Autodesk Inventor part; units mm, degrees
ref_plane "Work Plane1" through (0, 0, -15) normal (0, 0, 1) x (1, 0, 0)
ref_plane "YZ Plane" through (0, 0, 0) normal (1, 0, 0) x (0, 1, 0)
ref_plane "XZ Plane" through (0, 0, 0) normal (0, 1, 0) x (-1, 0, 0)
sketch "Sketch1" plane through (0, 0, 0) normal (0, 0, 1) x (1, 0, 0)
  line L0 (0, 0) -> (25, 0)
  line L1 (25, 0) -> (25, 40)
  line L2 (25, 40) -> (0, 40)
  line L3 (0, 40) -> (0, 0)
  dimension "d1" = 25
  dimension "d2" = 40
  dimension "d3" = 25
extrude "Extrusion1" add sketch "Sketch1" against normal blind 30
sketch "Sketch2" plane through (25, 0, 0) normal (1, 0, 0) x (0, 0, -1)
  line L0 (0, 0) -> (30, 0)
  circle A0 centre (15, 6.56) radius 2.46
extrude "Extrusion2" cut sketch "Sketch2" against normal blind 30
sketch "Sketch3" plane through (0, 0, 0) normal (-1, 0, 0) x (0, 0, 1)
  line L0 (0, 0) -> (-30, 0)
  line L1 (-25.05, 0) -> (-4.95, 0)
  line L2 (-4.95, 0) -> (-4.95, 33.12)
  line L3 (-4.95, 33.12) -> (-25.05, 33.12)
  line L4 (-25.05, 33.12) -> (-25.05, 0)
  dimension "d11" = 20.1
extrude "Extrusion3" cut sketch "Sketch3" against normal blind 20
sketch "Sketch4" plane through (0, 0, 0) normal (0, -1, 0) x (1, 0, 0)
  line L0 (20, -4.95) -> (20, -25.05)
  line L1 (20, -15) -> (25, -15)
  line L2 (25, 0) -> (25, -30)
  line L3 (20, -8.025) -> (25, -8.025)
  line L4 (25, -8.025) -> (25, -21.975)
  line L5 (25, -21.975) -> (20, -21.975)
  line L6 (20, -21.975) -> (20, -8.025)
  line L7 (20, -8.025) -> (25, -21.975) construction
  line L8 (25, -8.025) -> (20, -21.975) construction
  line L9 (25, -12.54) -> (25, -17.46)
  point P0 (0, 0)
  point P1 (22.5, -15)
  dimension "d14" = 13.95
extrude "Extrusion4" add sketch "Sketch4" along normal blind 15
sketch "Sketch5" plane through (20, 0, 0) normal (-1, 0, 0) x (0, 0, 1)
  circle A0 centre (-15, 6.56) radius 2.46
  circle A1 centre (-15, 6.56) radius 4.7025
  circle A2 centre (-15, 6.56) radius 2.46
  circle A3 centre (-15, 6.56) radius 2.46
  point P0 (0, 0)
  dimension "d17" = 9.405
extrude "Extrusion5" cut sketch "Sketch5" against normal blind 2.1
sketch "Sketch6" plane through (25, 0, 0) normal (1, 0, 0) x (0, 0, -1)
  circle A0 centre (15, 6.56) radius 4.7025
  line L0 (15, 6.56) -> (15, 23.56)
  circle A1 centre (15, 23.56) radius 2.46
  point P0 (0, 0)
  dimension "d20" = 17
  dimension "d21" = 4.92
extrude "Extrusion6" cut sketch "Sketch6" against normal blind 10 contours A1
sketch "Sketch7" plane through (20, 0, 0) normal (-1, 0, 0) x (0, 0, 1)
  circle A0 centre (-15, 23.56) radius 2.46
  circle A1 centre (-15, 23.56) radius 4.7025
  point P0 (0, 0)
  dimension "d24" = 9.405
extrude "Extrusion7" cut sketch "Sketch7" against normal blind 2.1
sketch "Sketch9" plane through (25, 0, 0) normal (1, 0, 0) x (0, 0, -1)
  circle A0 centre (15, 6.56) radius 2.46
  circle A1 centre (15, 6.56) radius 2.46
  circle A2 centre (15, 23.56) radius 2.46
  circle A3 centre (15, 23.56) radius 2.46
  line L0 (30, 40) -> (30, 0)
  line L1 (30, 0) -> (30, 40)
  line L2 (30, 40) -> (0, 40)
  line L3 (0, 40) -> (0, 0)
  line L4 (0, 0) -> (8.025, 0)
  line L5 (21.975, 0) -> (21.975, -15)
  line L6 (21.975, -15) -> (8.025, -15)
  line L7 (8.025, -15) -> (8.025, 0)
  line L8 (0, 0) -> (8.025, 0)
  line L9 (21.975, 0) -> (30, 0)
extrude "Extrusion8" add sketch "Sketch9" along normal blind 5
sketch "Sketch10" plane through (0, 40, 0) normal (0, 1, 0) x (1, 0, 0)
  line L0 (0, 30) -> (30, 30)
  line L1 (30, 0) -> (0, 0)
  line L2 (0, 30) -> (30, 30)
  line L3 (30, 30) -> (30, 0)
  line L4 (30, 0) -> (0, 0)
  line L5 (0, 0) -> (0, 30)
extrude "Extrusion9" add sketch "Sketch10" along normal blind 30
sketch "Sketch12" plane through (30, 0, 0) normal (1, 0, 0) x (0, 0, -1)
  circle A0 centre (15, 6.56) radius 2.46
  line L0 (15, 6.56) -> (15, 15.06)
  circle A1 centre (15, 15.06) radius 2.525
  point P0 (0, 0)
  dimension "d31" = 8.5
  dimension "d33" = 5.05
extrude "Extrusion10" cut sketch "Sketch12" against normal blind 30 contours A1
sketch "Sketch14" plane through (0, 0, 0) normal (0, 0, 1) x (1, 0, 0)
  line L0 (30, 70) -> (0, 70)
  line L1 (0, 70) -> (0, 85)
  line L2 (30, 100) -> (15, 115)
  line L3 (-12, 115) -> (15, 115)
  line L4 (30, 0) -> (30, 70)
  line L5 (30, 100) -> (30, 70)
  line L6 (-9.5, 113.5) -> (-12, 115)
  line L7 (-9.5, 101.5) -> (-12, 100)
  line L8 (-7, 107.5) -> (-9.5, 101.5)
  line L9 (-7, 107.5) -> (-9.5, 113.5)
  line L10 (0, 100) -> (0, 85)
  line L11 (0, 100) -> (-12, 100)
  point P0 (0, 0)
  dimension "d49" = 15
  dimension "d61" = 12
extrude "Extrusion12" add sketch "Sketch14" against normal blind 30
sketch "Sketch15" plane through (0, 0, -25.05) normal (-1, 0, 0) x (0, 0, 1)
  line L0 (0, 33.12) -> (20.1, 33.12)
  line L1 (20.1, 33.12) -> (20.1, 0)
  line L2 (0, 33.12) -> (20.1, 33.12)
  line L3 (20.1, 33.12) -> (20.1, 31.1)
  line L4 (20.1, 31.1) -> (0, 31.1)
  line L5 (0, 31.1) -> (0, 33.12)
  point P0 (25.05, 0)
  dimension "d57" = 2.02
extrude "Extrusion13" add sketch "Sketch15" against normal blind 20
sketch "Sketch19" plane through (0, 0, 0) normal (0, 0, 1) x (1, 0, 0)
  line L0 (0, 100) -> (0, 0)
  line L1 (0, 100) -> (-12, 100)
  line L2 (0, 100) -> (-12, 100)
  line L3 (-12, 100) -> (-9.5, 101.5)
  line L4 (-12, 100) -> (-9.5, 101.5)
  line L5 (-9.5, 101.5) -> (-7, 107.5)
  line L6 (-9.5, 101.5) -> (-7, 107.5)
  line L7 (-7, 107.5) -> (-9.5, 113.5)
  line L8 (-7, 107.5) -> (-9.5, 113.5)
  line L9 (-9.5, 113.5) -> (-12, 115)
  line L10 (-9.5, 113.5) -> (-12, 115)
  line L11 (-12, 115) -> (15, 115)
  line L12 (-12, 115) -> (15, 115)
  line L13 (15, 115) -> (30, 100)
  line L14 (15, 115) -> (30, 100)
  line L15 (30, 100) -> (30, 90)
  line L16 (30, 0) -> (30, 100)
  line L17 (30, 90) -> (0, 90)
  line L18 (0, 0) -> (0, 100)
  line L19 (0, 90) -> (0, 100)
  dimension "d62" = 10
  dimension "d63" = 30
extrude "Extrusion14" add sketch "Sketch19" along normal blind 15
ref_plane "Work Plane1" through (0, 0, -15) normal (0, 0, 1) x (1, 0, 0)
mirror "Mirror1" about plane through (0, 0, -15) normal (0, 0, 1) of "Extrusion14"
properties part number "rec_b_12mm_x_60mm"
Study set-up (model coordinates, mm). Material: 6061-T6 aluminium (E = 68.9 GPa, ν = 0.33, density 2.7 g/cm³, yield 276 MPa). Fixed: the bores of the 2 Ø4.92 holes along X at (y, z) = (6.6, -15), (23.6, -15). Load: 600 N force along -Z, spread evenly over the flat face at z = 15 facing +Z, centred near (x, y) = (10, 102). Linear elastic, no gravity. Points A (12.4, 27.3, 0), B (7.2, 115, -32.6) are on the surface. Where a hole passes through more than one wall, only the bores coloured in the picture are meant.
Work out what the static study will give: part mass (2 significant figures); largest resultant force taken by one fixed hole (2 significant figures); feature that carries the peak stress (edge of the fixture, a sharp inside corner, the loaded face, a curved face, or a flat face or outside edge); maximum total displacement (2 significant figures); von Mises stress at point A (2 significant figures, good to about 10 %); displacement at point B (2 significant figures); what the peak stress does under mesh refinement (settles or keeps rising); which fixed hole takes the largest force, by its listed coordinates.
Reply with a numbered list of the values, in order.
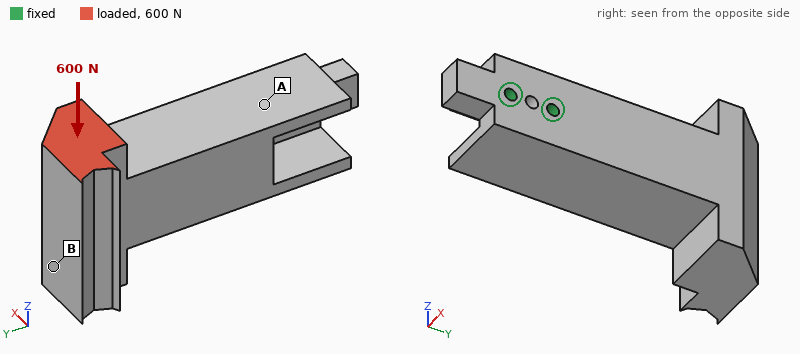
1. 310 g
2. 2.6 kN
3. edge of the fixture
4. 100 µm
5. 13 MPa
6. 91 µm
7. keeps rising
8. (23.6, -15)
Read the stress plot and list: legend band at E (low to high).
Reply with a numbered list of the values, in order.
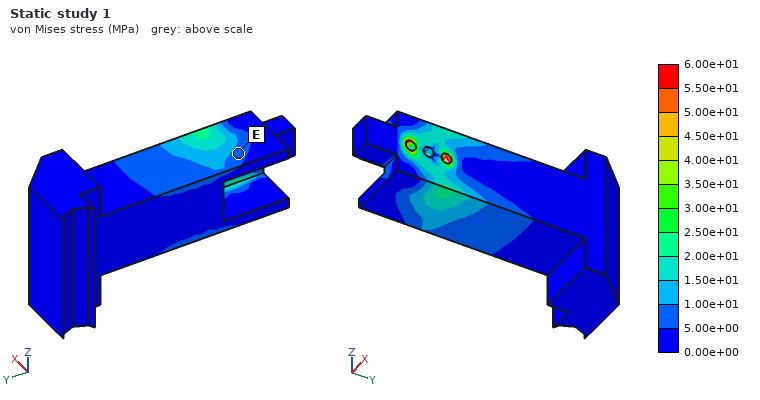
1. 5.00e+00 to 1.00e+01 MPa
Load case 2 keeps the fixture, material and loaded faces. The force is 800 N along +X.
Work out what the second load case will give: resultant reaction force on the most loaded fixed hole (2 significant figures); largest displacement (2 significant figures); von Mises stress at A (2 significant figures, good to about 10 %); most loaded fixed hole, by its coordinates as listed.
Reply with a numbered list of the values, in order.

1. 3.3 kN
2. 0.22 mm
3. 17 MPa
4. (23.6, -15)
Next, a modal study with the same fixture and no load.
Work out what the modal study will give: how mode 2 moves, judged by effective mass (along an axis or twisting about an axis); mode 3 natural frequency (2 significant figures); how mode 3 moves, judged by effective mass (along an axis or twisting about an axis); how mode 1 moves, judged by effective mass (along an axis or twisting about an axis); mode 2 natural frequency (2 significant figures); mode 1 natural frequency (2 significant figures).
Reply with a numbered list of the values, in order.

1. along Z
2. 2300 Hz
3. twisting about Y
4. along X
5. 1100 Hz
6. 940 Hz
